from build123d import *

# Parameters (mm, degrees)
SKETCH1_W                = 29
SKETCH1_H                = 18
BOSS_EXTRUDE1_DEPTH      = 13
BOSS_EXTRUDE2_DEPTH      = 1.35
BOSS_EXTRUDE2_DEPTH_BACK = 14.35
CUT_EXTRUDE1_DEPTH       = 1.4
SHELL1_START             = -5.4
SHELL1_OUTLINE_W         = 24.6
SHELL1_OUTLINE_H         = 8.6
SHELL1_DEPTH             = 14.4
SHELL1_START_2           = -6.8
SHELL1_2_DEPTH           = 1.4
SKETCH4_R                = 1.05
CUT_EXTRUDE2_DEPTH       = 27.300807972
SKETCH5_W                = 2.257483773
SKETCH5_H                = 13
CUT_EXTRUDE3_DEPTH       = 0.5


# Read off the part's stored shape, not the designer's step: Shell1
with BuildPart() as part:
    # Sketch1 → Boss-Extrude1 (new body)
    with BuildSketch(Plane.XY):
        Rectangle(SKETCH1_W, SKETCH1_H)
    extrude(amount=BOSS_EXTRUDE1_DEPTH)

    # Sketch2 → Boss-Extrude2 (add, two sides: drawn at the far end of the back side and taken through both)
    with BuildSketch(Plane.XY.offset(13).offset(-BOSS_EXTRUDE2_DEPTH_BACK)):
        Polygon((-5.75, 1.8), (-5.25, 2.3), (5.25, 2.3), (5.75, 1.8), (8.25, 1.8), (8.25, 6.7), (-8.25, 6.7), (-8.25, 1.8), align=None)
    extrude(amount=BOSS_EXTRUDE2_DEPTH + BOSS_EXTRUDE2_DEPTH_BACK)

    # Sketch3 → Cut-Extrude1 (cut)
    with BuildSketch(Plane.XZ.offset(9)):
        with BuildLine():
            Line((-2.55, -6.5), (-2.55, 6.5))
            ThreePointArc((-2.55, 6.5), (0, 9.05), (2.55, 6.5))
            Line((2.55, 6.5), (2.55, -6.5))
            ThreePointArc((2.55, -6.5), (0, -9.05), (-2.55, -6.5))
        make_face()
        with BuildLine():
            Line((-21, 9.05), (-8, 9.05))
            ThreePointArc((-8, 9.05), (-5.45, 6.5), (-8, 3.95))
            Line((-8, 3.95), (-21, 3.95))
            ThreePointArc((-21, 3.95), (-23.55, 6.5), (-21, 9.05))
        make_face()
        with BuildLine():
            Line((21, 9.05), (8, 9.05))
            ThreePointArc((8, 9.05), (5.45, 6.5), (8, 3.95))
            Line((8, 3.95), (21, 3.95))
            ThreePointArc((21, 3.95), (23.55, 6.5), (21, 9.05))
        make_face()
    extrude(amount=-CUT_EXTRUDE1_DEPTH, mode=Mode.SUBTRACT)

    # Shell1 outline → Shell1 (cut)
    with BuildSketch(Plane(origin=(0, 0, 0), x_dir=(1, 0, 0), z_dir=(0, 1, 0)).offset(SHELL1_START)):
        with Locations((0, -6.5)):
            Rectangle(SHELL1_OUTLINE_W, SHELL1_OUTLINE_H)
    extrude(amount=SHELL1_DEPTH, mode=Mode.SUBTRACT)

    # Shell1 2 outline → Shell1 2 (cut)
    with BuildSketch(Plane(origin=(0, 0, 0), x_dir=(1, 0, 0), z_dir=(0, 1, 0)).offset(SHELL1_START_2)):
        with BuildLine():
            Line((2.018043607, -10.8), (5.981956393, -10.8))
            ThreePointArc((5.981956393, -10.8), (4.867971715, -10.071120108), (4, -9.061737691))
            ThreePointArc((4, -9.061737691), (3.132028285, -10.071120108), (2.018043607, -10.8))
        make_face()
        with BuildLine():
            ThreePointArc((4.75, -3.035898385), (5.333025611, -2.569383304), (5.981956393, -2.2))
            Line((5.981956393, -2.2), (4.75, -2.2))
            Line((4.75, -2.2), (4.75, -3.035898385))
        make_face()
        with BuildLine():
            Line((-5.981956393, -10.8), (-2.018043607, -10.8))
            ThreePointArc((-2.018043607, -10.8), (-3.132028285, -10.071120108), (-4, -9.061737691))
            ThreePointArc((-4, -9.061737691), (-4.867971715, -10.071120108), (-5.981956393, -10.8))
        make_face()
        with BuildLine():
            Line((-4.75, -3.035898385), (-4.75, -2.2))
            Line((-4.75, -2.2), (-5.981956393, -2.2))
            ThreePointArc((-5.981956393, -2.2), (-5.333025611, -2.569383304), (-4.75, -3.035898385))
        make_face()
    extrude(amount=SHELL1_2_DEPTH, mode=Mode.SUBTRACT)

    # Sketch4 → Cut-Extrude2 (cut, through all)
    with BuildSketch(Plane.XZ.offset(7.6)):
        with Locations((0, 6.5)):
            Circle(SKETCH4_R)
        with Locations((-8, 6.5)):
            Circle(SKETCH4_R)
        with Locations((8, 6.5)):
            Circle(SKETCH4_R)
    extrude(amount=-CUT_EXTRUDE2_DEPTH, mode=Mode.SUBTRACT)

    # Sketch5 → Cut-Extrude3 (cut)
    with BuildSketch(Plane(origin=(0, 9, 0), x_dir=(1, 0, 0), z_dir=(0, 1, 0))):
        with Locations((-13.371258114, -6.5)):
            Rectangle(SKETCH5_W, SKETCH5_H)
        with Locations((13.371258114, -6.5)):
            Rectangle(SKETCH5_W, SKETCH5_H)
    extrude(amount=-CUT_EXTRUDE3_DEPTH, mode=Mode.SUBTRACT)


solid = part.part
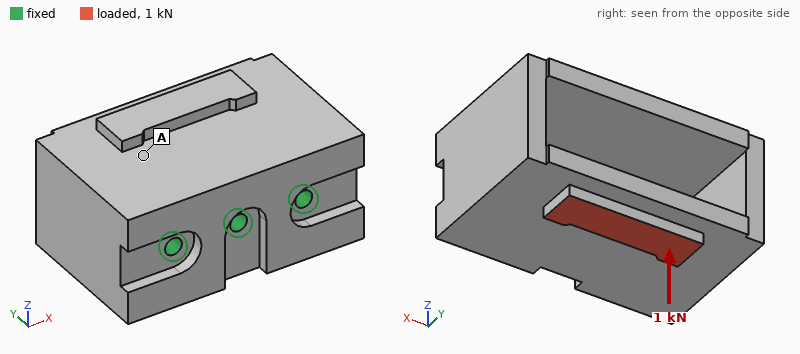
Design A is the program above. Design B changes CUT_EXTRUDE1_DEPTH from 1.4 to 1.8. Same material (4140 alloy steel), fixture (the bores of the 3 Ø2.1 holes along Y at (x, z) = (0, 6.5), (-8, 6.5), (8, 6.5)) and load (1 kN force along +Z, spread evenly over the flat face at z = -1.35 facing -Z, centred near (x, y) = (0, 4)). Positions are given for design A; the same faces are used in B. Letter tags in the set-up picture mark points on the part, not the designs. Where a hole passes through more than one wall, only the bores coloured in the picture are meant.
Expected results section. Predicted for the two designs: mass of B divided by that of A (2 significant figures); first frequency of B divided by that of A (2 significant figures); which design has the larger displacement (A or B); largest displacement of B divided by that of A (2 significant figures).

0.99
0.86
B
1.2
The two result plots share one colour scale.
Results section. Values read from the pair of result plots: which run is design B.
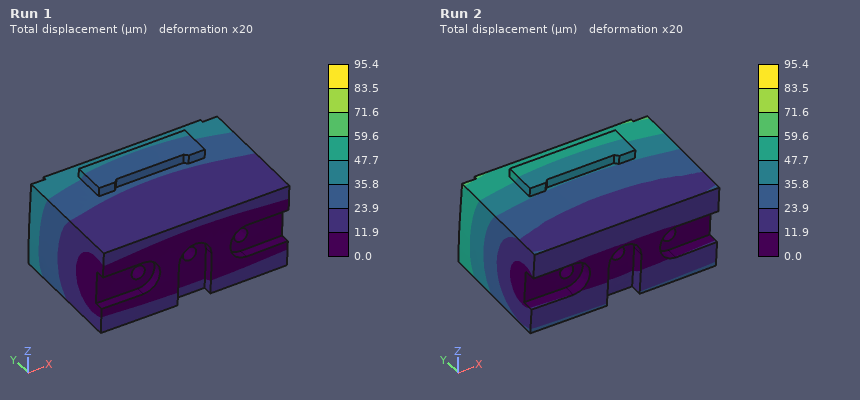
Run 2
